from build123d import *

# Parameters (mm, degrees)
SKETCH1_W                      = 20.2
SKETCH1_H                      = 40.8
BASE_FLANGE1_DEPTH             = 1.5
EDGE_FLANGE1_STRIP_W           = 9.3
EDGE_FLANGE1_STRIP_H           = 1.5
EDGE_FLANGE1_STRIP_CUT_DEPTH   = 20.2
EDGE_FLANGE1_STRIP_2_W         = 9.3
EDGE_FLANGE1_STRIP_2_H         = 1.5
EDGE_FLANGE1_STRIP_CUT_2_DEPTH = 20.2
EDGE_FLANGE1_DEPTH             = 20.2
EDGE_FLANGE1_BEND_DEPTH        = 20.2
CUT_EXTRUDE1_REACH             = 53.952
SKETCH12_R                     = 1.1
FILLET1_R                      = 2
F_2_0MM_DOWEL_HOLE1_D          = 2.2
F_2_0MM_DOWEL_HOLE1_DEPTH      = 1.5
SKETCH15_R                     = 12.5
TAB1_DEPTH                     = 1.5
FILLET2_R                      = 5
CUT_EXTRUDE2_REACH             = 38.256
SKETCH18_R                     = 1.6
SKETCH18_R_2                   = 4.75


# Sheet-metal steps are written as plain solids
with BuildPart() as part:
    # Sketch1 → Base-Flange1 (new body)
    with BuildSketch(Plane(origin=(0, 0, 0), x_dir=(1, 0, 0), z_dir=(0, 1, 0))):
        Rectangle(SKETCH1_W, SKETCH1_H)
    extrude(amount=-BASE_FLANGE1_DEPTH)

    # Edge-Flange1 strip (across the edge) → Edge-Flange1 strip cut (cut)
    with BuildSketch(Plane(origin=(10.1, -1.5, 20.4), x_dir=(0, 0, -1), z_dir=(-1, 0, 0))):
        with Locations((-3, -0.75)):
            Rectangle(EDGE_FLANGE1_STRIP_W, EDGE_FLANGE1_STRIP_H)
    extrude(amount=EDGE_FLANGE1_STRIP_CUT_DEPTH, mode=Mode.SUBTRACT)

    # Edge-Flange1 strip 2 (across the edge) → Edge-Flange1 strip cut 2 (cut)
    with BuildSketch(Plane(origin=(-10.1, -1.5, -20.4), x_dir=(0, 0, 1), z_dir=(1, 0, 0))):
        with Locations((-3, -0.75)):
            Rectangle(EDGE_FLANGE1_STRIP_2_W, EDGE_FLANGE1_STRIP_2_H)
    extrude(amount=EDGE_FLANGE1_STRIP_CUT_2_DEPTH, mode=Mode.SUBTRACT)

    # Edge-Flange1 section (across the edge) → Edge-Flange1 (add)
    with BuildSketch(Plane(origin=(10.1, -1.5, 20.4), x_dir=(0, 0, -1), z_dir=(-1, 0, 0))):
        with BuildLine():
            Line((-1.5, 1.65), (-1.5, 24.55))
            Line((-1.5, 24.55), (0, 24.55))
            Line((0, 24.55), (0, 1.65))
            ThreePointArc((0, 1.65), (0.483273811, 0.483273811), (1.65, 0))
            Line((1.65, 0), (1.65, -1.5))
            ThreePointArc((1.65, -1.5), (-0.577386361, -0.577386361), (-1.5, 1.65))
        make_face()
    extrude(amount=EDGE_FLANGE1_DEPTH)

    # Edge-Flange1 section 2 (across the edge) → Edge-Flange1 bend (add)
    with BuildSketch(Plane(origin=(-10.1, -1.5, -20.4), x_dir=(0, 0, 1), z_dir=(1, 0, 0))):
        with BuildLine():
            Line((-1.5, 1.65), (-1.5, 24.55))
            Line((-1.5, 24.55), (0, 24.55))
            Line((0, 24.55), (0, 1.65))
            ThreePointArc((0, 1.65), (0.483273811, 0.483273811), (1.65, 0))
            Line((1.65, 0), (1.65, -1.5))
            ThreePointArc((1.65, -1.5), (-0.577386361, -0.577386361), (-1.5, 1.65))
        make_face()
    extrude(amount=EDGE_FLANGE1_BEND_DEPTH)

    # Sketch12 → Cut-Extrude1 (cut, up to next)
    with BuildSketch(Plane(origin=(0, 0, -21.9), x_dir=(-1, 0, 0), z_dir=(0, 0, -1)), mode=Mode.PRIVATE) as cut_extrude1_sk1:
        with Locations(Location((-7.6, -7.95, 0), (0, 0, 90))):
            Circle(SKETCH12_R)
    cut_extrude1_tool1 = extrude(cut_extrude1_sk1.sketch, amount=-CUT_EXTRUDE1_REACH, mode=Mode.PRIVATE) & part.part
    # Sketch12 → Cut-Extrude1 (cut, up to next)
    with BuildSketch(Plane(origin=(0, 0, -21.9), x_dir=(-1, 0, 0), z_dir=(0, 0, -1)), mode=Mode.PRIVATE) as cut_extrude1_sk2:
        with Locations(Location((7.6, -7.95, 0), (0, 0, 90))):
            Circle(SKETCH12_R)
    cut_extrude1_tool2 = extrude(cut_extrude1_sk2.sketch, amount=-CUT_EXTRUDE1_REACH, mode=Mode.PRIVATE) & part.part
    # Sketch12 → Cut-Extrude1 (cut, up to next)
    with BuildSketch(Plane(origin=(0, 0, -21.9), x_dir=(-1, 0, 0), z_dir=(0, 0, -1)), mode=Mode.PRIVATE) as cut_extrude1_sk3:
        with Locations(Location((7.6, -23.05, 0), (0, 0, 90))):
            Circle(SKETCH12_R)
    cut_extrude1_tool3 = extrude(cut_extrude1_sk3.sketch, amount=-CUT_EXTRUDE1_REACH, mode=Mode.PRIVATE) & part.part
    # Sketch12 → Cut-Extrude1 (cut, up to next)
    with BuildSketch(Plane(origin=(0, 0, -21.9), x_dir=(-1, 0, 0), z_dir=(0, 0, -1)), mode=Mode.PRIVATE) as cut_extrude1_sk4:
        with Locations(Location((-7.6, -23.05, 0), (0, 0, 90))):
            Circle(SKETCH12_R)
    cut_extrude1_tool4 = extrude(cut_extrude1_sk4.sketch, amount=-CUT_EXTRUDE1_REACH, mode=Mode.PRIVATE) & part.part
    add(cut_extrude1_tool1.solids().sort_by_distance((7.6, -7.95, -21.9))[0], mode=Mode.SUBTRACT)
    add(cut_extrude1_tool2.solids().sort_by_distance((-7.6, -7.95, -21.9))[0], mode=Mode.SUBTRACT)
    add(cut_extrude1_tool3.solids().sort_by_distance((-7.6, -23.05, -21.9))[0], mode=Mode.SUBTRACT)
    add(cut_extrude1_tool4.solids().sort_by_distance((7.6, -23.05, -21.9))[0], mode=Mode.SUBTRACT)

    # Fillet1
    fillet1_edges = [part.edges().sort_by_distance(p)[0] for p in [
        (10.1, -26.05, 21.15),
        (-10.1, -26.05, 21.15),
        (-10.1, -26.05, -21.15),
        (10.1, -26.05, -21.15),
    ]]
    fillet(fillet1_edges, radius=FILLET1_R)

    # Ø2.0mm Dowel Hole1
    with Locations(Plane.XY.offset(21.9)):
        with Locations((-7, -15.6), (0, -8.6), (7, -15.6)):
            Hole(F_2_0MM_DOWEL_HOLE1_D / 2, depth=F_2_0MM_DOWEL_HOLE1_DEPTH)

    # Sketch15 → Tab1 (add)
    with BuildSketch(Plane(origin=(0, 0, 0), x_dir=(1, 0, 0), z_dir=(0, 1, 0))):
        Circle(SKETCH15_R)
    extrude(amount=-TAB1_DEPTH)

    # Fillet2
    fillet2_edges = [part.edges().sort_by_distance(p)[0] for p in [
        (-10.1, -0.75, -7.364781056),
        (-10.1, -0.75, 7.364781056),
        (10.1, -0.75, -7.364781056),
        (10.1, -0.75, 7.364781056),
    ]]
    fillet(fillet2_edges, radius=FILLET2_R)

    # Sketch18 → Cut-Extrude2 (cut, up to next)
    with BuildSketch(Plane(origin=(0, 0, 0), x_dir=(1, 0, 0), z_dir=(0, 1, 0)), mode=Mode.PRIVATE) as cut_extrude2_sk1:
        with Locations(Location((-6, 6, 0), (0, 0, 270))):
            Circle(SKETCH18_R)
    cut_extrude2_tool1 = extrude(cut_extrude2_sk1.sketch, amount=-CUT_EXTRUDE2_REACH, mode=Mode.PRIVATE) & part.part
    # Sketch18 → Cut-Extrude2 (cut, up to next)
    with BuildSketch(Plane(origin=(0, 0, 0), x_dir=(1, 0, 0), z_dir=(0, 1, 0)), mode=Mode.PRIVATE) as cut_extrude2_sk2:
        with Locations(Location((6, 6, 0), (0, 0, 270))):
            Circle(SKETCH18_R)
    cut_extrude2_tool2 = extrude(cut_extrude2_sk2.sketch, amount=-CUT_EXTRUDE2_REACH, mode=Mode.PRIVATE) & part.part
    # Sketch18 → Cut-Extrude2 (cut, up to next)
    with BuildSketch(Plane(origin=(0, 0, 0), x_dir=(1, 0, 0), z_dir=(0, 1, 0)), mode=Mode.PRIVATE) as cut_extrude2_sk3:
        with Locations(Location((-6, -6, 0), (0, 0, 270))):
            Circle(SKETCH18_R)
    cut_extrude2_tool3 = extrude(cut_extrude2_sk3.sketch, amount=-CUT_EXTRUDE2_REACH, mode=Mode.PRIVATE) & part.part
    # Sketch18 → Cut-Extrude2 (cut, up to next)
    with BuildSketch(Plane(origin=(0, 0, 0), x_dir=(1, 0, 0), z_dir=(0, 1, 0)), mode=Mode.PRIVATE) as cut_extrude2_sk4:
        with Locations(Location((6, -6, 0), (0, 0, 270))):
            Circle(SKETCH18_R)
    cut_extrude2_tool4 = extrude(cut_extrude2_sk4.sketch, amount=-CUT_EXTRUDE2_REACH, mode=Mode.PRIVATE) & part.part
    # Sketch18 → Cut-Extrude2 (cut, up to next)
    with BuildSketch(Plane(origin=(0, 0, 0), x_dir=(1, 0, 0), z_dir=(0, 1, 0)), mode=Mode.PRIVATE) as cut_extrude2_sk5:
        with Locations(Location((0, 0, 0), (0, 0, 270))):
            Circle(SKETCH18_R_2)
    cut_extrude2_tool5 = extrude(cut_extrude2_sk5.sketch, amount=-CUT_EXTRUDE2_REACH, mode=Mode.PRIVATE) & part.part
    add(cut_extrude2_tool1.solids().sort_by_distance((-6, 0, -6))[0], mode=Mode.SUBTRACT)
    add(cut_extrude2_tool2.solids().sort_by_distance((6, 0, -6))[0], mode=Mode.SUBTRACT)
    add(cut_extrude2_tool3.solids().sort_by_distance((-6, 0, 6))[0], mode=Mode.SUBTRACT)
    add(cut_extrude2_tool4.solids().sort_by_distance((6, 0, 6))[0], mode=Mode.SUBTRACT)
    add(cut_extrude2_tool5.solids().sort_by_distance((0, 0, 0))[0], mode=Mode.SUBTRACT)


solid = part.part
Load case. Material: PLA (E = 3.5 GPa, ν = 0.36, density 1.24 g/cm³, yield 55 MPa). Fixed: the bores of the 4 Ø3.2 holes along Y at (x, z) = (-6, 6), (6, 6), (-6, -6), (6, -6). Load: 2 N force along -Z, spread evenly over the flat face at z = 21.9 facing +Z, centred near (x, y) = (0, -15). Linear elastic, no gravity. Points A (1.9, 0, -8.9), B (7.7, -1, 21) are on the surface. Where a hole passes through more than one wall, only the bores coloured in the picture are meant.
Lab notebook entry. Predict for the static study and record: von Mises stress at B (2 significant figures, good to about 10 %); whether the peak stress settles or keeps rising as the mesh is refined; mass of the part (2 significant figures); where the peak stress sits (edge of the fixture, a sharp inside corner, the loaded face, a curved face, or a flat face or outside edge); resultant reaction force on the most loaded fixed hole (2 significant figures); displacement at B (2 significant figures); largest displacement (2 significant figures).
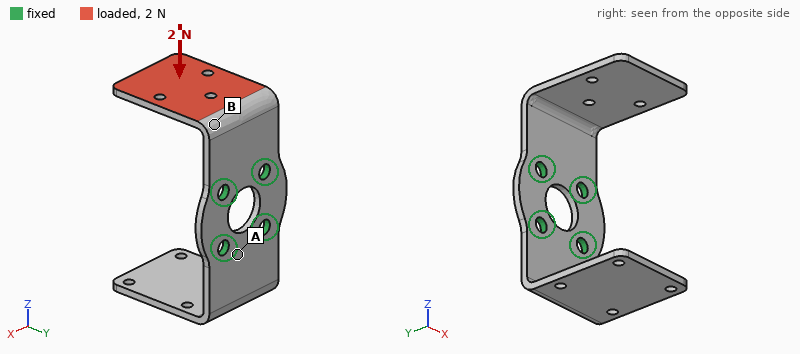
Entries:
2.5 MPa
keeps rising
3.3 g
edge of the fixture
1.0 N
0.13 mm
0.66 mm
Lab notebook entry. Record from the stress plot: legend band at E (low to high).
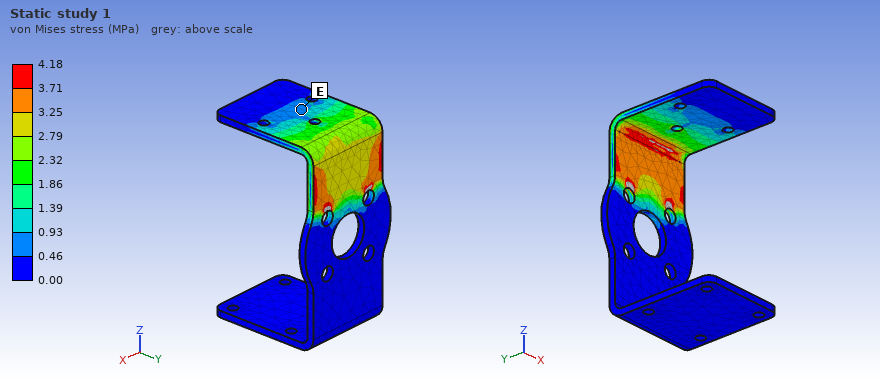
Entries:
0.46 to 0.93 MPa
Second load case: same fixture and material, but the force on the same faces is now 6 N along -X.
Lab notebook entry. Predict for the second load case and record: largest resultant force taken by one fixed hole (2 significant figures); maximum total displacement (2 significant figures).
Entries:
8.9 N
0.57 mm
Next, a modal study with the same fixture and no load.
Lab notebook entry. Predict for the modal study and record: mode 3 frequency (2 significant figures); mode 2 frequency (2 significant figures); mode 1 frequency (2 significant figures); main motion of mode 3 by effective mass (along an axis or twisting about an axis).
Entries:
640 Hz
350 Hz
350 Hz
along X
